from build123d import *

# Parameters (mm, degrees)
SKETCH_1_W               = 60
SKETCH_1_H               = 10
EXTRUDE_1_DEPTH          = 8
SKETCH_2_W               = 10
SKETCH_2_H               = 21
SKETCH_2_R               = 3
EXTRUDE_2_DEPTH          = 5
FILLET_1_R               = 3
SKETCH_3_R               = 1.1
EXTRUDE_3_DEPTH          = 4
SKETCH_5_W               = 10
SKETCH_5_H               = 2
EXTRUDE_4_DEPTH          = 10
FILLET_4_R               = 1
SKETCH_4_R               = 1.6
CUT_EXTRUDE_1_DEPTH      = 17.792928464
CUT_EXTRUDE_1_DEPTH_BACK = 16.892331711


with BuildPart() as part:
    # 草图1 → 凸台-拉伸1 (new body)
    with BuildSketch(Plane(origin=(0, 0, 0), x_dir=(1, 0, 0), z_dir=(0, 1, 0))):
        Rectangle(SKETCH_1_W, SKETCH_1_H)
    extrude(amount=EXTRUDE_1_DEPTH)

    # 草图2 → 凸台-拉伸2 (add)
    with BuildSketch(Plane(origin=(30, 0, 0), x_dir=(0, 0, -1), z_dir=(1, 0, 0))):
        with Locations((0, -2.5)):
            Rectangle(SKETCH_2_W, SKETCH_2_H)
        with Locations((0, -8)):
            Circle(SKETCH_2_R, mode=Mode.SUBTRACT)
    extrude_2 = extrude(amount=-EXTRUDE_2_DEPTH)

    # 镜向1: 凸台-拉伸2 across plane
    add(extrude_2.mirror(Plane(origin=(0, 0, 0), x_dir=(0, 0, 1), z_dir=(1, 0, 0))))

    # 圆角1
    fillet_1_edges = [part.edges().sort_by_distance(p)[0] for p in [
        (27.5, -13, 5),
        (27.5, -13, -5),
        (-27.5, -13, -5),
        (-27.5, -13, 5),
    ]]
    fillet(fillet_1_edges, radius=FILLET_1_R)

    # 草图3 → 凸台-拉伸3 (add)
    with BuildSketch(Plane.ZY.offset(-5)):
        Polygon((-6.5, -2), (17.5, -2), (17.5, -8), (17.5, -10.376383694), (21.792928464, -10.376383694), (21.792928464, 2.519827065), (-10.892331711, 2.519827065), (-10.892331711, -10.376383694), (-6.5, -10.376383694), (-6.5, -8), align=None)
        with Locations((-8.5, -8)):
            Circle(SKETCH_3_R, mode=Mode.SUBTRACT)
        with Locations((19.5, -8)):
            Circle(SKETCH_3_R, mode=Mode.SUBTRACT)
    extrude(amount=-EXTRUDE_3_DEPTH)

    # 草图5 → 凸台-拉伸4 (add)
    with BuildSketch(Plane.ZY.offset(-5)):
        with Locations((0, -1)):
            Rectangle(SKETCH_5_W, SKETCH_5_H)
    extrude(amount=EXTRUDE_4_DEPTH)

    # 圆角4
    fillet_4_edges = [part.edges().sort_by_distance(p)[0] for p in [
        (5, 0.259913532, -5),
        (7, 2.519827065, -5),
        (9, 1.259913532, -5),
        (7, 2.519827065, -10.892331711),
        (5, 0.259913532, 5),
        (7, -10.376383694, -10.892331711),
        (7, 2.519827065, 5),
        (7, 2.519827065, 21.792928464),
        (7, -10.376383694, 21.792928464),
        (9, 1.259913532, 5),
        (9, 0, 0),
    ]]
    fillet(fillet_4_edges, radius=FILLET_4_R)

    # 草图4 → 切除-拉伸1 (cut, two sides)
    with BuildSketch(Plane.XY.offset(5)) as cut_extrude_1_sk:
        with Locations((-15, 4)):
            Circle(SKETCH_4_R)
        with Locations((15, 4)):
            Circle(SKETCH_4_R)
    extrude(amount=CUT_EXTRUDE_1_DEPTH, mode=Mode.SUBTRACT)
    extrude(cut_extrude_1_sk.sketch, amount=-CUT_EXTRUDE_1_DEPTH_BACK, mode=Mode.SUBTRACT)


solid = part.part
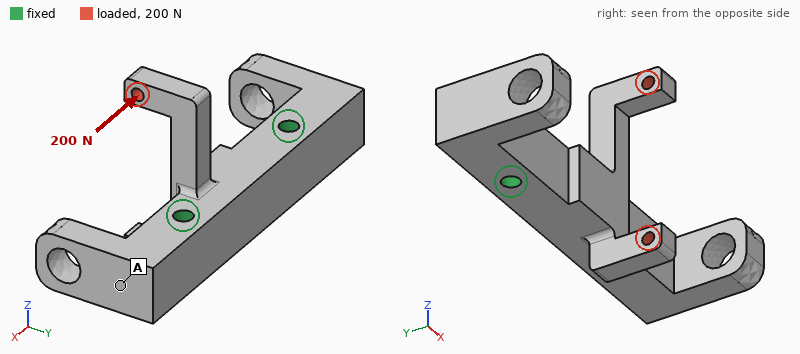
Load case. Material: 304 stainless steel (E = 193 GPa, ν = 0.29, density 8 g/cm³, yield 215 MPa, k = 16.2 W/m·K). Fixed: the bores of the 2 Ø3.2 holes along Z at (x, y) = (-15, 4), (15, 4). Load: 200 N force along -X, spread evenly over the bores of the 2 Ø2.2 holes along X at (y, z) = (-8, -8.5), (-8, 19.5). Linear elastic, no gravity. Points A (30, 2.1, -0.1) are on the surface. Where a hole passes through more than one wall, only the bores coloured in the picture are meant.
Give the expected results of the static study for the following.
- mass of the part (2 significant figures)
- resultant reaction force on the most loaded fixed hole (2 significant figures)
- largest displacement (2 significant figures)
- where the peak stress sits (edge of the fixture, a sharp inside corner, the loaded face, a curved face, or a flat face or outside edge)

53 g
150 N
72 µm
a curved face
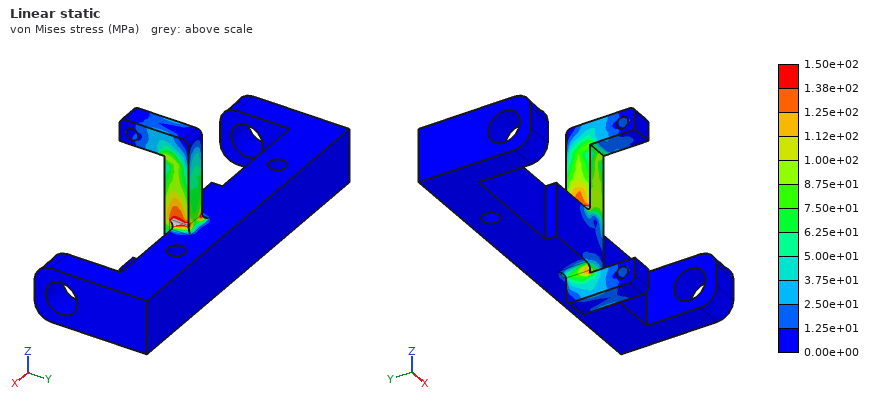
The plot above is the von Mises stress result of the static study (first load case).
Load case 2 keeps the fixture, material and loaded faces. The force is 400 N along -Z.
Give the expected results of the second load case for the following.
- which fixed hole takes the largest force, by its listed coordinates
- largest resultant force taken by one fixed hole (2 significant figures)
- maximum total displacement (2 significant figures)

(15, 4)
320 N
80 µm
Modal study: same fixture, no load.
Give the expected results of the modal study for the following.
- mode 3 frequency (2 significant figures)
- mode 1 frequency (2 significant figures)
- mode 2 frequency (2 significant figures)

11 kHz
6100 Hz
6300 Hz
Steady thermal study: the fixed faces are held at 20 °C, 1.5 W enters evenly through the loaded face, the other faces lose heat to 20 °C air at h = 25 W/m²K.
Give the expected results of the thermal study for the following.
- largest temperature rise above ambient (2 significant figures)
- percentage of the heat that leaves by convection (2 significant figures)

49 K
32 %
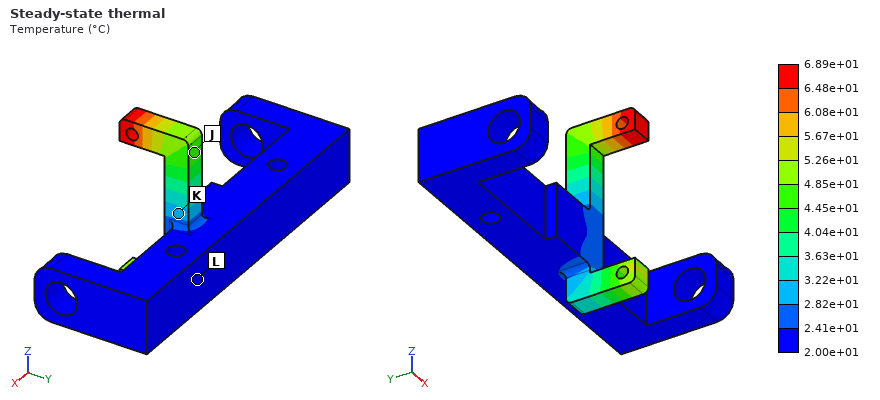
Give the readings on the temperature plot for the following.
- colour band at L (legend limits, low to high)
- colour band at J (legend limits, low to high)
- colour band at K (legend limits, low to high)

2.00e+01 to 2.41e+01 °C
4.45e+01 to 4.85e+01 °C
2.82e+01 to 3.22e+01 °C
